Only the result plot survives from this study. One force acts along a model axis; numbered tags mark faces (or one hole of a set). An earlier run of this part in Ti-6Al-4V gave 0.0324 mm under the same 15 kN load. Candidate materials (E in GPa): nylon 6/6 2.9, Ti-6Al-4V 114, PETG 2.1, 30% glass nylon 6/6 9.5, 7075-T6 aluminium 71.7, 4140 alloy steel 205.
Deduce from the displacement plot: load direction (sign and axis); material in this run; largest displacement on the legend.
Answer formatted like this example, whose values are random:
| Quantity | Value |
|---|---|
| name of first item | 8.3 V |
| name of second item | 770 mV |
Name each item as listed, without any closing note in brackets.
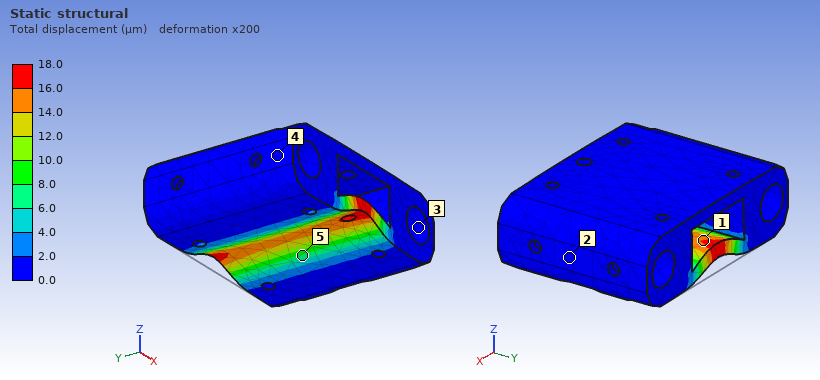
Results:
| Quantity | Value |
|---|---|
| load direction | +Z |
| material in this run | 4140 alloy steel |
| largest displacement on the legend | 18.0 µm |
